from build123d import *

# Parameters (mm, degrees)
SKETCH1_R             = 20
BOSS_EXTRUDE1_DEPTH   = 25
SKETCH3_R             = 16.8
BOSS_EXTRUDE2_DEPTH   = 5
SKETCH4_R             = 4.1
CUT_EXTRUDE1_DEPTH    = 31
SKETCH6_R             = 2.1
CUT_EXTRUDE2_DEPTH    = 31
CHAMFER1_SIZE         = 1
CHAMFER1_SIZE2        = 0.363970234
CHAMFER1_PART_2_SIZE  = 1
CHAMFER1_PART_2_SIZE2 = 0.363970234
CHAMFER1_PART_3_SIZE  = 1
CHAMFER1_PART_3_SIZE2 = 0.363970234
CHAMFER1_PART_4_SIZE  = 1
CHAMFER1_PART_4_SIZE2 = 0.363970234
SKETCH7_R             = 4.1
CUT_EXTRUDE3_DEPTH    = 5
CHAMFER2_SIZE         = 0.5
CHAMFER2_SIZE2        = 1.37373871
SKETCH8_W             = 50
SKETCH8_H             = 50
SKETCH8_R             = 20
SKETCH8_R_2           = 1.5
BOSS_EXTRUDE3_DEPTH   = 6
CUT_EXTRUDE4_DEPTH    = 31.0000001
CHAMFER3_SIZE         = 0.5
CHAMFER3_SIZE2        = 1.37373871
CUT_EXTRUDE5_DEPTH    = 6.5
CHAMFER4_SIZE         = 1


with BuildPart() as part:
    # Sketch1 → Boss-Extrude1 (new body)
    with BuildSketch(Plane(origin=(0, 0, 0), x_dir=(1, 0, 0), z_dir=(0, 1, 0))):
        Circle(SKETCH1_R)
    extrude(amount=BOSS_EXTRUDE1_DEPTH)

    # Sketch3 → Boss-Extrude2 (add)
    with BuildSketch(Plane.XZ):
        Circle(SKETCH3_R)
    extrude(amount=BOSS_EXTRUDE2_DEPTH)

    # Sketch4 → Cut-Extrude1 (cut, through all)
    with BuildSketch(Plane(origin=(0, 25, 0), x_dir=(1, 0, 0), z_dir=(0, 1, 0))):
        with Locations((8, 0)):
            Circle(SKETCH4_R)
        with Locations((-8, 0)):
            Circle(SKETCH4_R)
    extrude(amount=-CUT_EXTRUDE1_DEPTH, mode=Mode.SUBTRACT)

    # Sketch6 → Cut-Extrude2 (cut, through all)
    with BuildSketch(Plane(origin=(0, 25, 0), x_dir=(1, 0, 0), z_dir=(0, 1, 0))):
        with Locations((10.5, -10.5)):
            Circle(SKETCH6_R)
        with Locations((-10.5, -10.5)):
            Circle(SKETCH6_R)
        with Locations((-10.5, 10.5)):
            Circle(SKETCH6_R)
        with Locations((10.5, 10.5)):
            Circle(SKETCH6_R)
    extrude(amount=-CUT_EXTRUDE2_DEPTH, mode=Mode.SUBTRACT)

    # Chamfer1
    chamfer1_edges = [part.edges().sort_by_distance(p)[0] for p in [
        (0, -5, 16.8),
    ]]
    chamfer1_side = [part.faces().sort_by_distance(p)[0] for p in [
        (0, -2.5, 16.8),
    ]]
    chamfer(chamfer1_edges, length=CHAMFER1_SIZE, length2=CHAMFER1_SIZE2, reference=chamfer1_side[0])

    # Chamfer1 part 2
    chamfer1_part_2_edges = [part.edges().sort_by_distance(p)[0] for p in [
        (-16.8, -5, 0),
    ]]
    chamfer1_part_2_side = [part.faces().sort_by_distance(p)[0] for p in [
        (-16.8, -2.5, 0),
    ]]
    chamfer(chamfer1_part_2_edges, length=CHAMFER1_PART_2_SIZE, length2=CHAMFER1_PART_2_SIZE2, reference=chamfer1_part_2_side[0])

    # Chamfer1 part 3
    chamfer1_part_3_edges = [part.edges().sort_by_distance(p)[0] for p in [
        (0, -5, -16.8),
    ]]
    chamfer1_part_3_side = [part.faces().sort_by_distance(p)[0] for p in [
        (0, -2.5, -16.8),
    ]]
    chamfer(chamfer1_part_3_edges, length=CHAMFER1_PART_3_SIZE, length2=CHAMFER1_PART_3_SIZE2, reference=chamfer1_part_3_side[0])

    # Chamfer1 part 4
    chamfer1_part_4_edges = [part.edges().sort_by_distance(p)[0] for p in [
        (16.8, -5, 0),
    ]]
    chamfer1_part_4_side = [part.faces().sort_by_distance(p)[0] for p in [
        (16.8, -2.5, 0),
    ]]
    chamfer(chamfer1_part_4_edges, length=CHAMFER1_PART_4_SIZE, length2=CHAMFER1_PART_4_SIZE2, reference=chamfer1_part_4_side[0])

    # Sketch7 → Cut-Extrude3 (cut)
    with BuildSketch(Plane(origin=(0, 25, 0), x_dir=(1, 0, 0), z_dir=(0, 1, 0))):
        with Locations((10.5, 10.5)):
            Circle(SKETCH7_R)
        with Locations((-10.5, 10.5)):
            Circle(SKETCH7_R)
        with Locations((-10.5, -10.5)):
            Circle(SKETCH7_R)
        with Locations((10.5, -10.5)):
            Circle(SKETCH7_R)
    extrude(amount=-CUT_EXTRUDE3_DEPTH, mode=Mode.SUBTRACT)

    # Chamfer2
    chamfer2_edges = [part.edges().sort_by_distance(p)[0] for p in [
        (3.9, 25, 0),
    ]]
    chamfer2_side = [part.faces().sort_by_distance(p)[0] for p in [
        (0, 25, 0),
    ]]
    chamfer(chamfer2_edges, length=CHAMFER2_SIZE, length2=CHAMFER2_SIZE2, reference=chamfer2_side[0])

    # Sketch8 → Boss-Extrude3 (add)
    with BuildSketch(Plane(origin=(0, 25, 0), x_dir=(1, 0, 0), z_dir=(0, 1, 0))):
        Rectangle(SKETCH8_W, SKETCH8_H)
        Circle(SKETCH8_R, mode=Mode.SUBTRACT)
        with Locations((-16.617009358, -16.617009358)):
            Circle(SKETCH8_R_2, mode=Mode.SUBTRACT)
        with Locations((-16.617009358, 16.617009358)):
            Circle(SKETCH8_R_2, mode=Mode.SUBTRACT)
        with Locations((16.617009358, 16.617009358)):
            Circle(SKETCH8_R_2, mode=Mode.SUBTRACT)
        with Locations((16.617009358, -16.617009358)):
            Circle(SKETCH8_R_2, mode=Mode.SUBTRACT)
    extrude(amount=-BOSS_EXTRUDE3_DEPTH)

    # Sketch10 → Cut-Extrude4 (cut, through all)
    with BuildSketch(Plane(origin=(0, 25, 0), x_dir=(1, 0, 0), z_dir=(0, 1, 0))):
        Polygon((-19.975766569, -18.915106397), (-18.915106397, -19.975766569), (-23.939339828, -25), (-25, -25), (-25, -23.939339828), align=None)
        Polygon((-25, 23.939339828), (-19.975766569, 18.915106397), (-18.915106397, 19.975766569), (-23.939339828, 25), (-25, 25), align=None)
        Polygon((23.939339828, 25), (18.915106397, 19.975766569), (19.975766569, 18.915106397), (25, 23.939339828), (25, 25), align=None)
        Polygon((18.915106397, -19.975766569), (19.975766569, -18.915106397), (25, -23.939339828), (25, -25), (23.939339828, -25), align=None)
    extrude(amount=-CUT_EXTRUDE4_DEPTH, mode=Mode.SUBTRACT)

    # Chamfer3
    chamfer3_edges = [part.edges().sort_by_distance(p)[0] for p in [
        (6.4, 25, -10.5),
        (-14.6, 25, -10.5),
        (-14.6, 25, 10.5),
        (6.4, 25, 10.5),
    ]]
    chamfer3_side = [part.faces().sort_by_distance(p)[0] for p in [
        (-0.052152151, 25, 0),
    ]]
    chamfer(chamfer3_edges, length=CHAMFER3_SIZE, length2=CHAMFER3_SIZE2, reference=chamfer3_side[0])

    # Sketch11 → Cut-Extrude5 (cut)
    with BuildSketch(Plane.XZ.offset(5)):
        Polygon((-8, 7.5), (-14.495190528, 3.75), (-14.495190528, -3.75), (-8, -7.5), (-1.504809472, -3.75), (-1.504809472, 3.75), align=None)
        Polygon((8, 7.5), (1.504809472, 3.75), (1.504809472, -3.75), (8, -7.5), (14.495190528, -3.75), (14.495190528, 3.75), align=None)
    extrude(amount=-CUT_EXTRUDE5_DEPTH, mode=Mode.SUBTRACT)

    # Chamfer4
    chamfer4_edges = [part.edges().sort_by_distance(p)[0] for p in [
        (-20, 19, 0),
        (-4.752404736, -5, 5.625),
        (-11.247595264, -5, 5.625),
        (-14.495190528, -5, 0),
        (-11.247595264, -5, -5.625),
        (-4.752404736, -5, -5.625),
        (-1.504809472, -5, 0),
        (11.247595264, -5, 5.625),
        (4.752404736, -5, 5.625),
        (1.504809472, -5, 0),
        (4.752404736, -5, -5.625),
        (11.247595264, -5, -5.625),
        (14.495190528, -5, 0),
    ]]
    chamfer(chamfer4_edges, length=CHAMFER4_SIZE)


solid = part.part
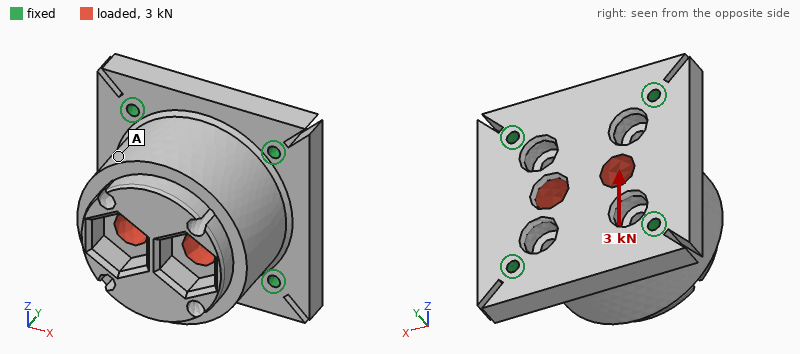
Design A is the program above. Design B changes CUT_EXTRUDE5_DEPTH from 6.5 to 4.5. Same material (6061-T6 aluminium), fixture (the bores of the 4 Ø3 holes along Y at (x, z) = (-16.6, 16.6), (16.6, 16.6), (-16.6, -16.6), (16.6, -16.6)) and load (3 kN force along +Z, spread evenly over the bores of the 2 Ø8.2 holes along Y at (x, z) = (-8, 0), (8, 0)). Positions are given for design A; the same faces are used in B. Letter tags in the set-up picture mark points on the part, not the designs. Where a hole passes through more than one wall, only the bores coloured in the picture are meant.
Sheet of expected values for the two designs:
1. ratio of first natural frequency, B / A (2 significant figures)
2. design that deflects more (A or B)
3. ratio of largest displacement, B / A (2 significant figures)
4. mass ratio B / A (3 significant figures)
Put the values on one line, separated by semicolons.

0.99; B; 1.1; 1.01
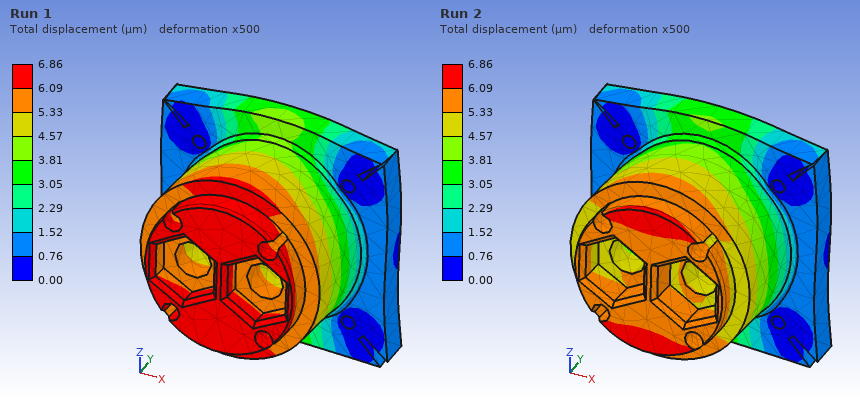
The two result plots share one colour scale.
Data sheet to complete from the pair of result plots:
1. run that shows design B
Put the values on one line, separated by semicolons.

Run 1
